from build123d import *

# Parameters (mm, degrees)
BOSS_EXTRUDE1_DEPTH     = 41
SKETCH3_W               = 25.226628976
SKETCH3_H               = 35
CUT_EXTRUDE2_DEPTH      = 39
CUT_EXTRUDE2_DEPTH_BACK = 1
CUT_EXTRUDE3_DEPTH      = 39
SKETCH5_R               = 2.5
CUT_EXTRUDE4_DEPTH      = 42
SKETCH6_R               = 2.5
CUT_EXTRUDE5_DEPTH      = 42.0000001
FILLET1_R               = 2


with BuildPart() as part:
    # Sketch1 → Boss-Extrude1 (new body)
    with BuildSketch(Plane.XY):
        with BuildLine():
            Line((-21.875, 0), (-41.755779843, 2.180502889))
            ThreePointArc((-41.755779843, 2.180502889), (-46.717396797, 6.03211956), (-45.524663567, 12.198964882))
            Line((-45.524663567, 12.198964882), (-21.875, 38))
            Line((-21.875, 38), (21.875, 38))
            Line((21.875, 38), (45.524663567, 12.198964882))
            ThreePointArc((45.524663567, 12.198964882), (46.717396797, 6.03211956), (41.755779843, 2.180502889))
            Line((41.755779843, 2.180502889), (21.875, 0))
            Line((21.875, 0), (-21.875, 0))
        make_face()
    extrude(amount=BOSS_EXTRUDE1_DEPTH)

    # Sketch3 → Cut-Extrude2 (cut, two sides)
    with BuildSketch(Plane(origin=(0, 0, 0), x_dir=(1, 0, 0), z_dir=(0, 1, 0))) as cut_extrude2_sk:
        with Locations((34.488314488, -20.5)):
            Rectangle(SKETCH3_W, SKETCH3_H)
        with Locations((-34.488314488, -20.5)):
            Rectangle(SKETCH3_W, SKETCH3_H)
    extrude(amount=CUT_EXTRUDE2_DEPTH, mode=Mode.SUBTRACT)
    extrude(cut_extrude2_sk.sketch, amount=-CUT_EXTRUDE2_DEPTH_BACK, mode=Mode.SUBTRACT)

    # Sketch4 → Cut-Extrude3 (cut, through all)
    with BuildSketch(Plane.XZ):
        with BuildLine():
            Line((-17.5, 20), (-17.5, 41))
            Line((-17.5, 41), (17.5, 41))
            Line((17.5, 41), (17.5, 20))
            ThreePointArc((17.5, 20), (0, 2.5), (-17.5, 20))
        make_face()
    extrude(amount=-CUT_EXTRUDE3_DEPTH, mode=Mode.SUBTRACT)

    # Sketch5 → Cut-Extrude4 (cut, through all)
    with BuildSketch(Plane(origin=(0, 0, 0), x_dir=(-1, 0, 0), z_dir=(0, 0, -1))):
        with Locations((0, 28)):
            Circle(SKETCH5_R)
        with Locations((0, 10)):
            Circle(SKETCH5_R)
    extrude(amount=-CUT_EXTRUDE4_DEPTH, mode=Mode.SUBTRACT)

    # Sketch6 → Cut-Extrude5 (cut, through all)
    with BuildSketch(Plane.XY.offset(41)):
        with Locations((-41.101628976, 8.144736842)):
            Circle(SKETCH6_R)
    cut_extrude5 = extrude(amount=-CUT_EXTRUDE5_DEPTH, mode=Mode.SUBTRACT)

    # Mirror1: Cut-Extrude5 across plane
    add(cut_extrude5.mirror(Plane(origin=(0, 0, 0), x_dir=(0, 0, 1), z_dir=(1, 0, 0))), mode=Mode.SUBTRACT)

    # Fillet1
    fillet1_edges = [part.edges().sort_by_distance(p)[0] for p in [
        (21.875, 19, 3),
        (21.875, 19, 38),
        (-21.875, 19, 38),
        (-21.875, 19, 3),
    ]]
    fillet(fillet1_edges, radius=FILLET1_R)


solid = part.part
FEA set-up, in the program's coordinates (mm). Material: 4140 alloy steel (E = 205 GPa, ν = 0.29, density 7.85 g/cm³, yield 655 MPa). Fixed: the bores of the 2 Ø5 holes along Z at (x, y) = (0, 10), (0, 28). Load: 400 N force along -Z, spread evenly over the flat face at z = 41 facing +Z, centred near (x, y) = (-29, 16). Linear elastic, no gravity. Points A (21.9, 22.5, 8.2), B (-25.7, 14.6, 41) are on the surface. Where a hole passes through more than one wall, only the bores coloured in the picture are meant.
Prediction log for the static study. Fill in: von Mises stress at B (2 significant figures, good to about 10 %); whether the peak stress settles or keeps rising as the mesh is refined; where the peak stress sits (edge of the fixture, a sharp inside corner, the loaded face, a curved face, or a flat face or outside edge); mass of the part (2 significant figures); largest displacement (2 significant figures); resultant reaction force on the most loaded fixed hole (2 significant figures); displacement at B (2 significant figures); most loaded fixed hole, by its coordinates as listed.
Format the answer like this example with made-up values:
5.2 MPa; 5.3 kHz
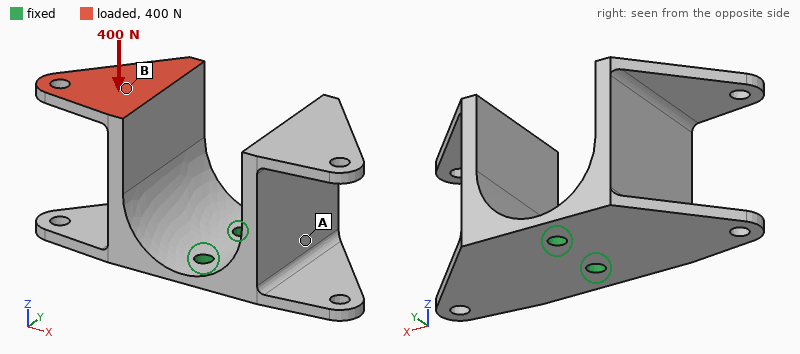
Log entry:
37 MPa; keeps rising; edge of the fixture; 220 g; 0.32 mm; 260 N; 0.21 mm; (0, 10)
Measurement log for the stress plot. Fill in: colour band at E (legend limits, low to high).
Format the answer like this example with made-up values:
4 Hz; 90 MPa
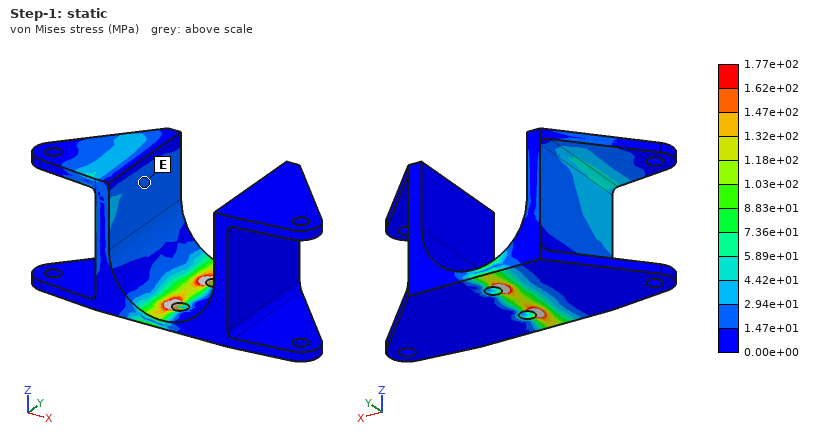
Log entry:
1.47e+01 to 2.94e+01 MPa
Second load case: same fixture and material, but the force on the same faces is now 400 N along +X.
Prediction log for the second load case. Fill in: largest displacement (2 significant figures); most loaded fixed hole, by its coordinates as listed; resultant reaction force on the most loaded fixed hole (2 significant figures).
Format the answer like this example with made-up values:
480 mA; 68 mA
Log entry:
0.49 mm; (0, 10); 270 N
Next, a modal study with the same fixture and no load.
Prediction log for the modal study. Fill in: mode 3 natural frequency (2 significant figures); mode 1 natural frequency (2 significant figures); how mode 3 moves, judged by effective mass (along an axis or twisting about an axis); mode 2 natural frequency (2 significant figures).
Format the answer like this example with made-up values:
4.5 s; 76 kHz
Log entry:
2600 Hz; 820 Hz; along Y; 840 Hz
